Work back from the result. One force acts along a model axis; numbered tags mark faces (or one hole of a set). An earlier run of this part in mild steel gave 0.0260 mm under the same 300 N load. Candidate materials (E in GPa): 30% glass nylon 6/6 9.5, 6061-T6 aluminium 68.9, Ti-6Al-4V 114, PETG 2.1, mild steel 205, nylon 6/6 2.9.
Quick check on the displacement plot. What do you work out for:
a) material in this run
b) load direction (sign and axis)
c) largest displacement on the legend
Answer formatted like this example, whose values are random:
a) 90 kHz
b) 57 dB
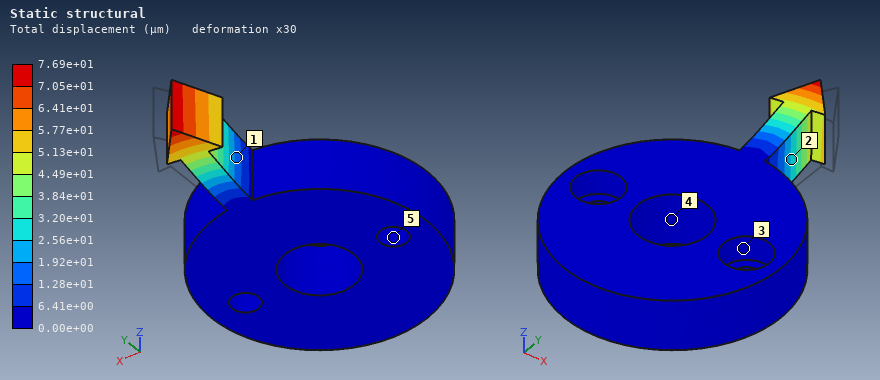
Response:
a) 6061-T6 aluminium
b) -X
c) 7.69e+01 µm
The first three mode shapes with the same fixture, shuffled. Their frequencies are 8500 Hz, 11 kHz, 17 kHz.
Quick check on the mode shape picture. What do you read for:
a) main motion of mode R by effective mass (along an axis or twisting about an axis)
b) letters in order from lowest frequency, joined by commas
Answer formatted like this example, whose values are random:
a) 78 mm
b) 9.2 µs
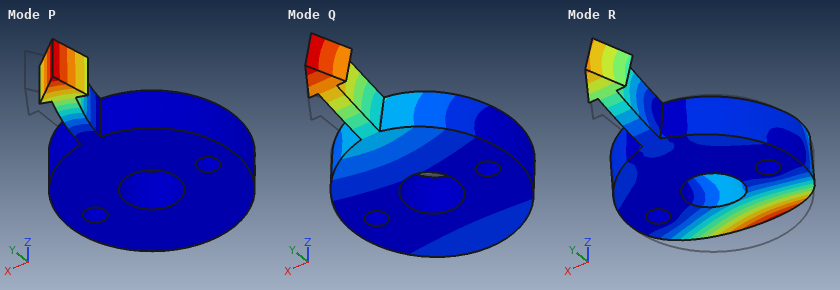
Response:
a) along Z
b) Q, P, R
